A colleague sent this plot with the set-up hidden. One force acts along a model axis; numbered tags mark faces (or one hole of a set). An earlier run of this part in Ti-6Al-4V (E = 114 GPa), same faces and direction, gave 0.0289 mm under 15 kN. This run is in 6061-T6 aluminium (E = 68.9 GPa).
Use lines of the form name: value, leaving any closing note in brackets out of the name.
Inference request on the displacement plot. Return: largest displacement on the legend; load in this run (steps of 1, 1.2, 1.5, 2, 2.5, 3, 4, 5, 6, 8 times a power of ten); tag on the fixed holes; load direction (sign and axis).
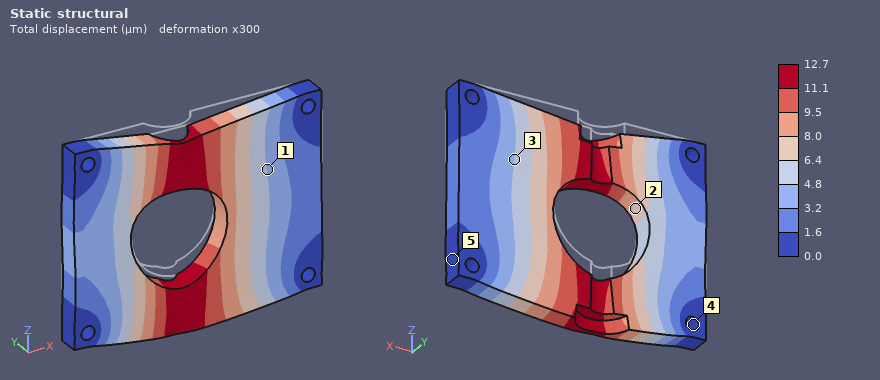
largest displacement on the legend: 12.7 µm
load in this run: 4 kN
tag on the fixed holes: 4
load direction: -Z
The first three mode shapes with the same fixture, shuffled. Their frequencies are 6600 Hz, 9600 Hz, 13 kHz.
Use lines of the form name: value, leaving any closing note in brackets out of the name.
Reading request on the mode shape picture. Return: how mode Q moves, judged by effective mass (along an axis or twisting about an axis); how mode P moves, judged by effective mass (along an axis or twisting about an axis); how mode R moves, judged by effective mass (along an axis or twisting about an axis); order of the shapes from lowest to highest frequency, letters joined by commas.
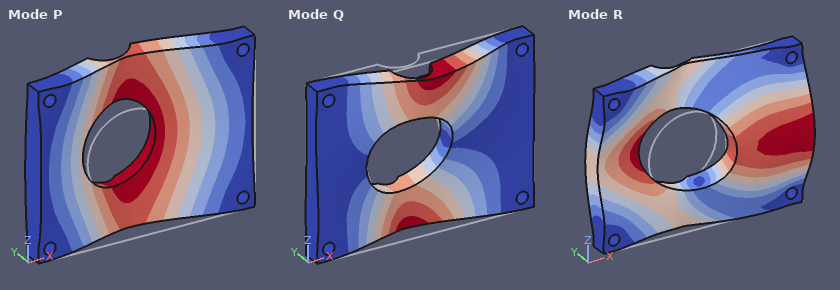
how mode Q moves, judged by effective mass: twisting about X
how mode P moves, judged by effective mass: along Y
how mode R moves, judged by effective mass: twisting about Z
order of the shapes from lowest to highest frequency, letters joined by commas: P, Q, R
